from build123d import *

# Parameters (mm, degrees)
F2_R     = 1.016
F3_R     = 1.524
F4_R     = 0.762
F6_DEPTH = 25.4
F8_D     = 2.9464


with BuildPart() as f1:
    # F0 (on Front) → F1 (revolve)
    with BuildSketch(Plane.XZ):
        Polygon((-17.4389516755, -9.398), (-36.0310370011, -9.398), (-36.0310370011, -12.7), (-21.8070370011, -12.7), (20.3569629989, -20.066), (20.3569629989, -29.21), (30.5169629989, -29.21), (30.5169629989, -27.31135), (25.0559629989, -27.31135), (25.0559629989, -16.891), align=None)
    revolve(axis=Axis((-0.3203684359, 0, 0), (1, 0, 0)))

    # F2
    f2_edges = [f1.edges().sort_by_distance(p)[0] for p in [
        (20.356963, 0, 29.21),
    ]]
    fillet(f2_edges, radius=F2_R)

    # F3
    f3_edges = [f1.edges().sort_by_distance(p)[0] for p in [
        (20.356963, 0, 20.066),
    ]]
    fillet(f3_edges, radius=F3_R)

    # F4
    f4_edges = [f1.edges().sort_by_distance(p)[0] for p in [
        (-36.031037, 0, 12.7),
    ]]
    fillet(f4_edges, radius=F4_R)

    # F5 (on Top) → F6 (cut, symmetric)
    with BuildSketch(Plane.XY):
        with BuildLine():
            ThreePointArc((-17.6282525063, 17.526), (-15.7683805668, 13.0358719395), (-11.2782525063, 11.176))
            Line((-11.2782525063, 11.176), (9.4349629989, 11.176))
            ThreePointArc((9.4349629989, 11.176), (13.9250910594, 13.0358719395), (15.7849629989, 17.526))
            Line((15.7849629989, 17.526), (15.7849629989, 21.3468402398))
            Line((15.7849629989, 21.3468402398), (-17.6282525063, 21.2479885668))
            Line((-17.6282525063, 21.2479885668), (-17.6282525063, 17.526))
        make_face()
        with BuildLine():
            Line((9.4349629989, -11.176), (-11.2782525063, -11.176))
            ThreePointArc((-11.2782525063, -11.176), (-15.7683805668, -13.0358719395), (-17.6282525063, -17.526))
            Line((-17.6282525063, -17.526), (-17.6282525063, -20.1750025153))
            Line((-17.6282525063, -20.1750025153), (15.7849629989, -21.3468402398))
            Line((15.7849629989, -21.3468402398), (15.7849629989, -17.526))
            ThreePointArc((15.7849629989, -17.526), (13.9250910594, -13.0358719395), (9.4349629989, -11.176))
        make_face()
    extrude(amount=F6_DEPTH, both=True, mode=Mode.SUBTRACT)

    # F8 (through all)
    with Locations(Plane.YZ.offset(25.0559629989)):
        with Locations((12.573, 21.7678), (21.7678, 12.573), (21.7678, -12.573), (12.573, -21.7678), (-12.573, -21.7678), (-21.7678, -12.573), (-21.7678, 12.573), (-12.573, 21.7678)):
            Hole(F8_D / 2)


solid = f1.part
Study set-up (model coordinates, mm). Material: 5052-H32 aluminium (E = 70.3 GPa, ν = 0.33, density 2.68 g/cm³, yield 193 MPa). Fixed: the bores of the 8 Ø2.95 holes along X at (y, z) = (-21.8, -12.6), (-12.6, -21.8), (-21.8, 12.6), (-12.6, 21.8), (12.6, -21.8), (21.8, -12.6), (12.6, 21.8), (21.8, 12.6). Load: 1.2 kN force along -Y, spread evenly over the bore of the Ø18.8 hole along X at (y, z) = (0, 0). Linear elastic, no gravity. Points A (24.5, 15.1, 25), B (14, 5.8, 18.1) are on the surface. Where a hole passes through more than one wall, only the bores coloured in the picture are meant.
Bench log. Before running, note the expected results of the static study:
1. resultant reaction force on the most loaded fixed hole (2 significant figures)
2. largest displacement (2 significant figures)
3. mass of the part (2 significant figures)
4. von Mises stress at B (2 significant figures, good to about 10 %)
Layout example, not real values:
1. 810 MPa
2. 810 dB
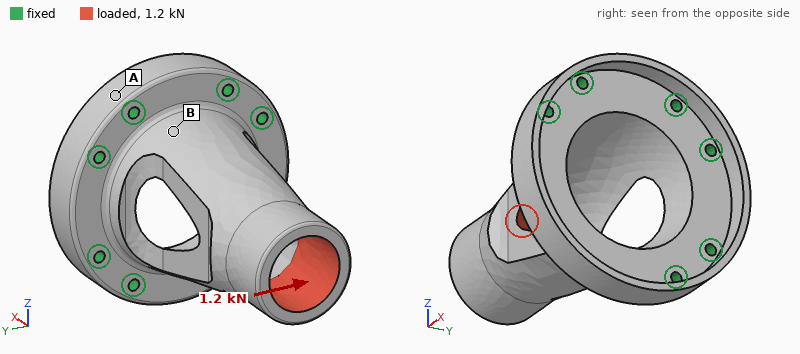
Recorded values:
1. 600 N
2. 0.11 mm
3. 65 g
4. 18 MPa
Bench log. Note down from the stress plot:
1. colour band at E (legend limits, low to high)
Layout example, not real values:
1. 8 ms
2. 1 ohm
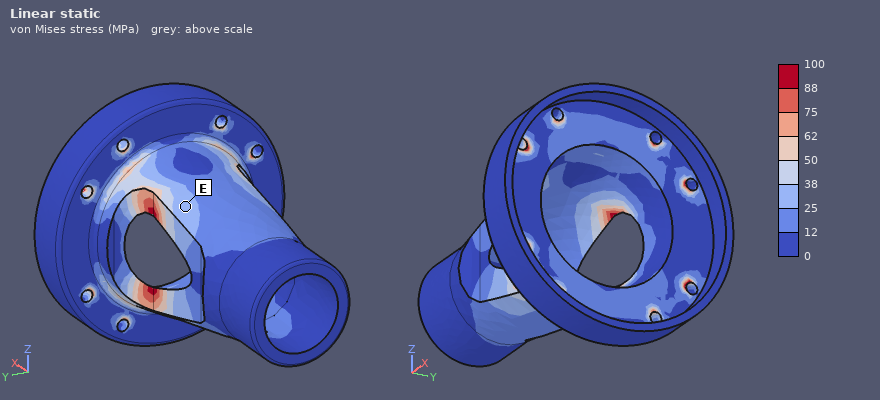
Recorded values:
1. 25 to 38 MPa
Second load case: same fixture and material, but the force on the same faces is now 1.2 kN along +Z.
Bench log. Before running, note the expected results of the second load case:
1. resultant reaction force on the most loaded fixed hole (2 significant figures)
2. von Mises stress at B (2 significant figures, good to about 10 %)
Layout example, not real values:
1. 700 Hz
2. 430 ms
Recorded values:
1. 750 N
2. 35 MPa
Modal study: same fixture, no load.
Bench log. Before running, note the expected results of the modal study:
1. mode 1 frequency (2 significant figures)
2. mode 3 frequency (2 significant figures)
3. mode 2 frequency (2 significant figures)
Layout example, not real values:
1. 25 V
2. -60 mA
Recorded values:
1. 4800 Hz
2. 11 kHz
3. 5000 Hz
